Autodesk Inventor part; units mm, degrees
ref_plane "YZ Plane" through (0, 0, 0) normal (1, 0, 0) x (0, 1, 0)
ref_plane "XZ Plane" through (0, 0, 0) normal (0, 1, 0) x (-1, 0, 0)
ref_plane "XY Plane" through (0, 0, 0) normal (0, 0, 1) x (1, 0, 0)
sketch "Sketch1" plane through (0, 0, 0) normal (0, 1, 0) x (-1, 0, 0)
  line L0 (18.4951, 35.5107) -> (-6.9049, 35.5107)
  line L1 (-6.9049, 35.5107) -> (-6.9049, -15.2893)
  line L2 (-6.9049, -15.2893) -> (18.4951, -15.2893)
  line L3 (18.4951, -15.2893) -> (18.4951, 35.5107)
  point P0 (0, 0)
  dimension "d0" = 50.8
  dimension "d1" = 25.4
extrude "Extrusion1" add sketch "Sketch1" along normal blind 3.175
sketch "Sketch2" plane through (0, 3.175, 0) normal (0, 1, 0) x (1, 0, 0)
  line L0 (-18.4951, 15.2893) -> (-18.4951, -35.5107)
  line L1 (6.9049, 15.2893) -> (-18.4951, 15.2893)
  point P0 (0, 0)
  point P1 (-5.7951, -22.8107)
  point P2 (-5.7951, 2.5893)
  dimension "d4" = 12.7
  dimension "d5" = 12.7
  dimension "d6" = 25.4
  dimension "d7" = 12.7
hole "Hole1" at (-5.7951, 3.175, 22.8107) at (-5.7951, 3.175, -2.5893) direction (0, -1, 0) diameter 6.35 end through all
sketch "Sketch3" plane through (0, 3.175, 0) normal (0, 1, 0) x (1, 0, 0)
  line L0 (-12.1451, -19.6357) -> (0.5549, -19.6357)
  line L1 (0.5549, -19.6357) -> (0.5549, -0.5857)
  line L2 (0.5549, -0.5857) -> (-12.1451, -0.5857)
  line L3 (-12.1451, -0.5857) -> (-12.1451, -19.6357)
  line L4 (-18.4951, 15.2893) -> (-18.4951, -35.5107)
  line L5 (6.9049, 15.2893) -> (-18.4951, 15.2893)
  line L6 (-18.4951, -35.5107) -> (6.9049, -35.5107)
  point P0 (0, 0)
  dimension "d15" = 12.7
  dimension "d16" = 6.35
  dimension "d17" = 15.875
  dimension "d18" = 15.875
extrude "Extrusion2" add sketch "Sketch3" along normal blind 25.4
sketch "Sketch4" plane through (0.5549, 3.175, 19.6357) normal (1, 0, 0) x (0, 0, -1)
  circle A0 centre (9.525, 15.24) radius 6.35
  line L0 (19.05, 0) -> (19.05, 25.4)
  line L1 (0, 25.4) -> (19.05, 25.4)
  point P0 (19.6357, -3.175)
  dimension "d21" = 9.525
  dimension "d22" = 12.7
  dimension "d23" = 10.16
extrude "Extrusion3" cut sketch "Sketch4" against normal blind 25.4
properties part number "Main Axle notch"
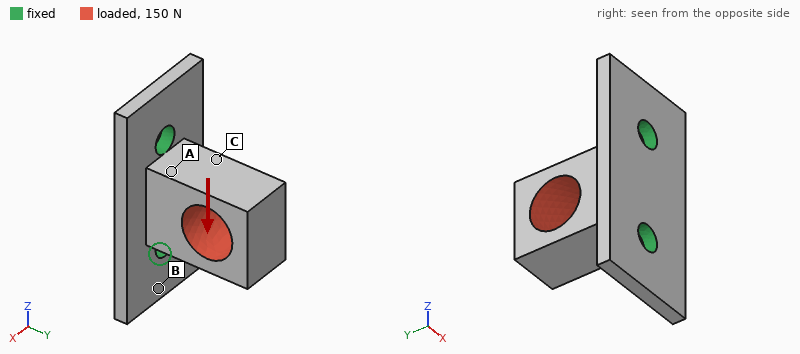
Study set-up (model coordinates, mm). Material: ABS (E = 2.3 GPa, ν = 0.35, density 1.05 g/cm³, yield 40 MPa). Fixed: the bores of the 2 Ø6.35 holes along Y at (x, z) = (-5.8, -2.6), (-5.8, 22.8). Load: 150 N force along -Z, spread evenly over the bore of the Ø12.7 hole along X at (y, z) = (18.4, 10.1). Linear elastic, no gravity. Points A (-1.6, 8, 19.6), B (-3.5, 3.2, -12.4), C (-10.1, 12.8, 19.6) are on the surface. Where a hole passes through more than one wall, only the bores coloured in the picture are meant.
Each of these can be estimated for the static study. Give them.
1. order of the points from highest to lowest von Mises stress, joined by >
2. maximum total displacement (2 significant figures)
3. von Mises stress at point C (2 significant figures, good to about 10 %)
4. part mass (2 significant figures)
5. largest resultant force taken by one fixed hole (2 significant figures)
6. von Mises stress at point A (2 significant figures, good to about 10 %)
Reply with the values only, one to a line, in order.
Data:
C > A > B
0.12 mm
4.2 MPa
8.9 g
150 N
3.1 MPa
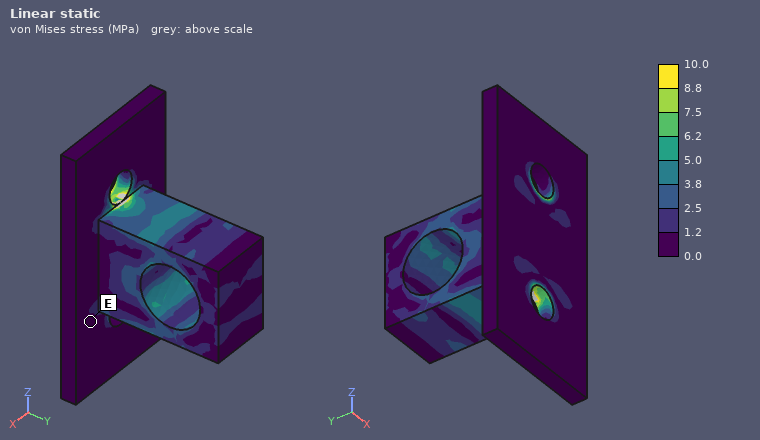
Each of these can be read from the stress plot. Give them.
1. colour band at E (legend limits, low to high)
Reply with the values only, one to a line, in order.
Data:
0.0 to 1.2 MPa
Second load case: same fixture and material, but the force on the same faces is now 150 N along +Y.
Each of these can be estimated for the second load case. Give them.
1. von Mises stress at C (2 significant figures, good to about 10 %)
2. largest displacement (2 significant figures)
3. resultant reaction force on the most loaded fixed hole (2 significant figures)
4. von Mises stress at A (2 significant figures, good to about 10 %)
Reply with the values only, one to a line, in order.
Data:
1.3 MPa
24 µm
80 N
1.5 MPa
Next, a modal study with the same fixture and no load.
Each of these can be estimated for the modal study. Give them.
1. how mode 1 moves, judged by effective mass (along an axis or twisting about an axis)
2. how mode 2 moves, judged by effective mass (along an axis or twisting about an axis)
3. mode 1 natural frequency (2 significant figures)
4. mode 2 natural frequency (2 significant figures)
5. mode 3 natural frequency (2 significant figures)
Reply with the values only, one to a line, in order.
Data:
along X
along Z
1800 Hz
3400 Hz
4900 Hz
